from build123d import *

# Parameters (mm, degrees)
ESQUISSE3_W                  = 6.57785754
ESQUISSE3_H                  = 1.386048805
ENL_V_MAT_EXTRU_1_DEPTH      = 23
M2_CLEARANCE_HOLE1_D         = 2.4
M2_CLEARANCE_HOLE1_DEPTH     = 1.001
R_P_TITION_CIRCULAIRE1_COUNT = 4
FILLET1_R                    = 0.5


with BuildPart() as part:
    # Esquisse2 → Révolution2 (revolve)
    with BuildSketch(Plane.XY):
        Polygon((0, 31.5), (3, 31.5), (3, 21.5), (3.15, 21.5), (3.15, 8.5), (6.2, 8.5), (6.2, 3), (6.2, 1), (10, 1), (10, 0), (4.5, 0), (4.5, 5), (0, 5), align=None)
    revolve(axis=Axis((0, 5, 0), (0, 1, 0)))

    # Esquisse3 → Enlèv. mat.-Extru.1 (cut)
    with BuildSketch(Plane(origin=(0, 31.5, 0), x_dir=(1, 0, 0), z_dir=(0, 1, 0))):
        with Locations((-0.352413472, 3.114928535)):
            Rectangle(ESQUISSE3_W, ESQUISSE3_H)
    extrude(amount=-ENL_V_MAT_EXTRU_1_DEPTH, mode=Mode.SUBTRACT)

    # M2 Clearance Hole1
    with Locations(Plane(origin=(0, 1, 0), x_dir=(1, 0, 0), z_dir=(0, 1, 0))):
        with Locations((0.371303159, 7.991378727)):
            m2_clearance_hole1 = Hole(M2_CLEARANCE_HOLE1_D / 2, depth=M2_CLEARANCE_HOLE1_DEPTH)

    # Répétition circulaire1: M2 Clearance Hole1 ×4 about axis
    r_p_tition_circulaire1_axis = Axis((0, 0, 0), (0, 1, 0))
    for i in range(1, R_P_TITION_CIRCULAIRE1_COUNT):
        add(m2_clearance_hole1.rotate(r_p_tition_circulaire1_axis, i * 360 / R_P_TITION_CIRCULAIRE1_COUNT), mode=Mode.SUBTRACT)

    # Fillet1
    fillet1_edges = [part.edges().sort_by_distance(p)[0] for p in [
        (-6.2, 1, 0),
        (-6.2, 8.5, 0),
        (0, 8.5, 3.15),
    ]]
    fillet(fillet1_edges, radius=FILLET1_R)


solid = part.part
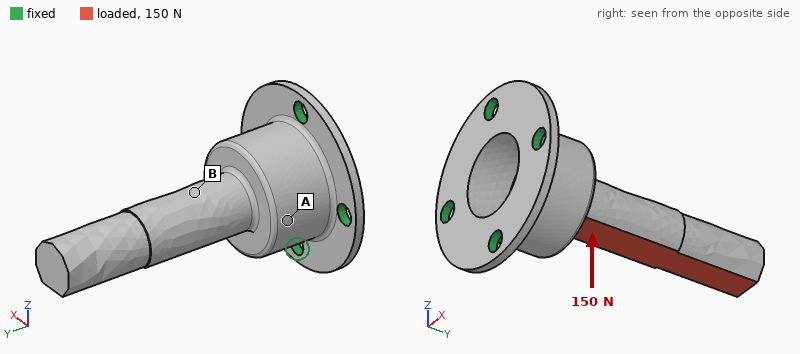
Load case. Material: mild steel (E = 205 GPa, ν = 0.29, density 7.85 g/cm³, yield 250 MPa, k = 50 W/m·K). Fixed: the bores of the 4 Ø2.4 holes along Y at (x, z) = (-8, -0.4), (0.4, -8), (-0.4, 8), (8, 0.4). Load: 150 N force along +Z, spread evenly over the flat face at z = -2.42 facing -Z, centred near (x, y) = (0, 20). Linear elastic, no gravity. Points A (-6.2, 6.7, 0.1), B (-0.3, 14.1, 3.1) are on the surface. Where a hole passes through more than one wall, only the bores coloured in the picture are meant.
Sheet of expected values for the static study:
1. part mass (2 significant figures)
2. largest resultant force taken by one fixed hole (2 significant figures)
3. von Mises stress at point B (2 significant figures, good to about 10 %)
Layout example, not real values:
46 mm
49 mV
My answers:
12 g
220 N
45 MPa
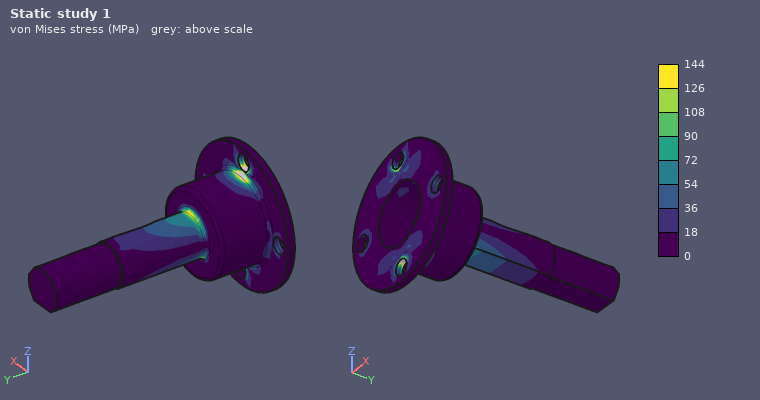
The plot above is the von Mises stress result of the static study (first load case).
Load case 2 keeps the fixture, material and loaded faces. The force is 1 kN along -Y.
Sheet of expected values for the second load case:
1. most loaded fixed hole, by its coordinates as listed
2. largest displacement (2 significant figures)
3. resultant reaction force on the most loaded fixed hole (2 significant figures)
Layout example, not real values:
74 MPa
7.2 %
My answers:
(0.4, -8)
53 µm
450 N
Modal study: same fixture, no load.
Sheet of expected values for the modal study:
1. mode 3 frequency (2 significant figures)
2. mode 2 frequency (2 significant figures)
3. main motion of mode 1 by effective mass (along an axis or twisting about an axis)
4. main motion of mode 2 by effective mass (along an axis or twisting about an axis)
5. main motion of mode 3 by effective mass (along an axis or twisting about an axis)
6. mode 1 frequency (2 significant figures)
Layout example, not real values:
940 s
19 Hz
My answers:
24 kHz
6300 Hz
along Z
along X
along Z
5900 Hz
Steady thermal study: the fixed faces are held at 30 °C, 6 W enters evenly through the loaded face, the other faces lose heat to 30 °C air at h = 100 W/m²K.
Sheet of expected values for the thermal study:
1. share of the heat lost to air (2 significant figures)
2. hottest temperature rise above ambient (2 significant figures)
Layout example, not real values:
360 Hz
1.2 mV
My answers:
37 %
51 K
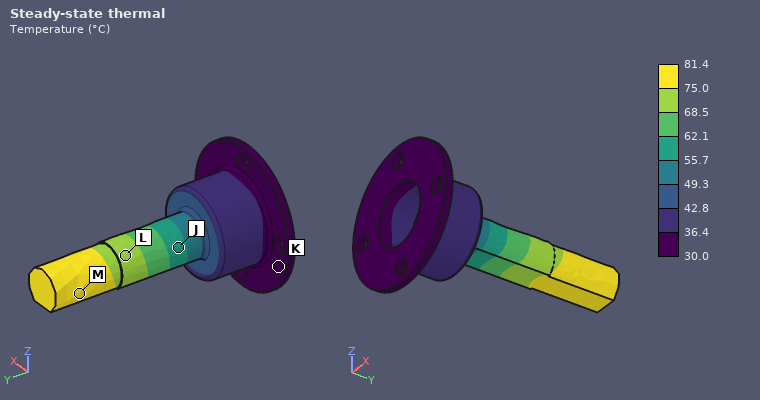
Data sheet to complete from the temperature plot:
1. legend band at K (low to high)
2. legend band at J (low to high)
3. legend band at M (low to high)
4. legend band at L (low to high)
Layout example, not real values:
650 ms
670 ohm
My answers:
30.0 to 36.4 °C
55.7 to 62.1 °C
75.0 to 81.4 °C
68.5 to 75.0 °C
